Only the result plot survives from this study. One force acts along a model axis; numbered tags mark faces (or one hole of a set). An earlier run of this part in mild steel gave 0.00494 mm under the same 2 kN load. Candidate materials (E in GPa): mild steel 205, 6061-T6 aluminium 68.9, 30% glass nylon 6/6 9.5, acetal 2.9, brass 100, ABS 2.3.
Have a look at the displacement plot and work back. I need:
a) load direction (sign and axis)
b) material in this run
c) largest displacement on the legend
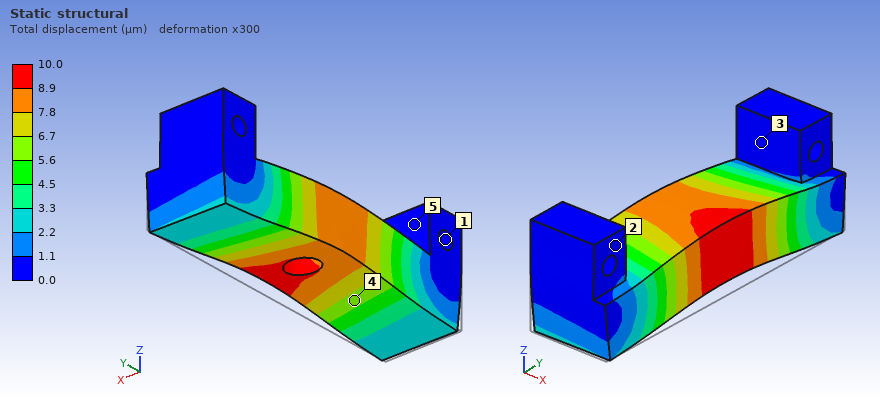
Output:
+Z
brass
10.0 µm
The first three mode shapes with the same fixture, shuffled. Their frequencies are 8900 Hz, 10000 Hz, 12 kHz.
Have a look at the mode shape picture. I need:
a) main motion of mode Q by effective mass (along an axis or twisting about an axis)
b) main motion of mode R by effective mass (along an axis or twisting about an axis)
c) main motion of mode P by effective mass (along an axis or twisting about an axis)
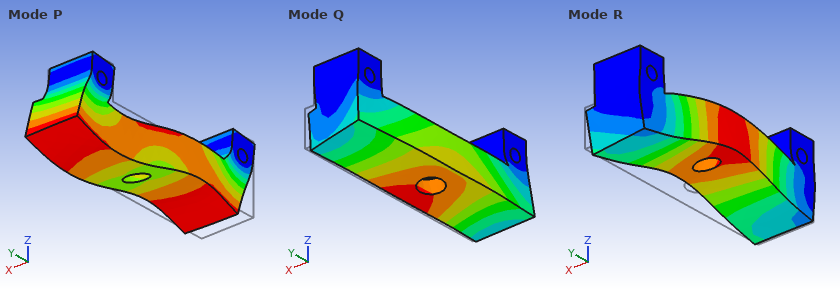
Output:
along X
along Z
along Y
